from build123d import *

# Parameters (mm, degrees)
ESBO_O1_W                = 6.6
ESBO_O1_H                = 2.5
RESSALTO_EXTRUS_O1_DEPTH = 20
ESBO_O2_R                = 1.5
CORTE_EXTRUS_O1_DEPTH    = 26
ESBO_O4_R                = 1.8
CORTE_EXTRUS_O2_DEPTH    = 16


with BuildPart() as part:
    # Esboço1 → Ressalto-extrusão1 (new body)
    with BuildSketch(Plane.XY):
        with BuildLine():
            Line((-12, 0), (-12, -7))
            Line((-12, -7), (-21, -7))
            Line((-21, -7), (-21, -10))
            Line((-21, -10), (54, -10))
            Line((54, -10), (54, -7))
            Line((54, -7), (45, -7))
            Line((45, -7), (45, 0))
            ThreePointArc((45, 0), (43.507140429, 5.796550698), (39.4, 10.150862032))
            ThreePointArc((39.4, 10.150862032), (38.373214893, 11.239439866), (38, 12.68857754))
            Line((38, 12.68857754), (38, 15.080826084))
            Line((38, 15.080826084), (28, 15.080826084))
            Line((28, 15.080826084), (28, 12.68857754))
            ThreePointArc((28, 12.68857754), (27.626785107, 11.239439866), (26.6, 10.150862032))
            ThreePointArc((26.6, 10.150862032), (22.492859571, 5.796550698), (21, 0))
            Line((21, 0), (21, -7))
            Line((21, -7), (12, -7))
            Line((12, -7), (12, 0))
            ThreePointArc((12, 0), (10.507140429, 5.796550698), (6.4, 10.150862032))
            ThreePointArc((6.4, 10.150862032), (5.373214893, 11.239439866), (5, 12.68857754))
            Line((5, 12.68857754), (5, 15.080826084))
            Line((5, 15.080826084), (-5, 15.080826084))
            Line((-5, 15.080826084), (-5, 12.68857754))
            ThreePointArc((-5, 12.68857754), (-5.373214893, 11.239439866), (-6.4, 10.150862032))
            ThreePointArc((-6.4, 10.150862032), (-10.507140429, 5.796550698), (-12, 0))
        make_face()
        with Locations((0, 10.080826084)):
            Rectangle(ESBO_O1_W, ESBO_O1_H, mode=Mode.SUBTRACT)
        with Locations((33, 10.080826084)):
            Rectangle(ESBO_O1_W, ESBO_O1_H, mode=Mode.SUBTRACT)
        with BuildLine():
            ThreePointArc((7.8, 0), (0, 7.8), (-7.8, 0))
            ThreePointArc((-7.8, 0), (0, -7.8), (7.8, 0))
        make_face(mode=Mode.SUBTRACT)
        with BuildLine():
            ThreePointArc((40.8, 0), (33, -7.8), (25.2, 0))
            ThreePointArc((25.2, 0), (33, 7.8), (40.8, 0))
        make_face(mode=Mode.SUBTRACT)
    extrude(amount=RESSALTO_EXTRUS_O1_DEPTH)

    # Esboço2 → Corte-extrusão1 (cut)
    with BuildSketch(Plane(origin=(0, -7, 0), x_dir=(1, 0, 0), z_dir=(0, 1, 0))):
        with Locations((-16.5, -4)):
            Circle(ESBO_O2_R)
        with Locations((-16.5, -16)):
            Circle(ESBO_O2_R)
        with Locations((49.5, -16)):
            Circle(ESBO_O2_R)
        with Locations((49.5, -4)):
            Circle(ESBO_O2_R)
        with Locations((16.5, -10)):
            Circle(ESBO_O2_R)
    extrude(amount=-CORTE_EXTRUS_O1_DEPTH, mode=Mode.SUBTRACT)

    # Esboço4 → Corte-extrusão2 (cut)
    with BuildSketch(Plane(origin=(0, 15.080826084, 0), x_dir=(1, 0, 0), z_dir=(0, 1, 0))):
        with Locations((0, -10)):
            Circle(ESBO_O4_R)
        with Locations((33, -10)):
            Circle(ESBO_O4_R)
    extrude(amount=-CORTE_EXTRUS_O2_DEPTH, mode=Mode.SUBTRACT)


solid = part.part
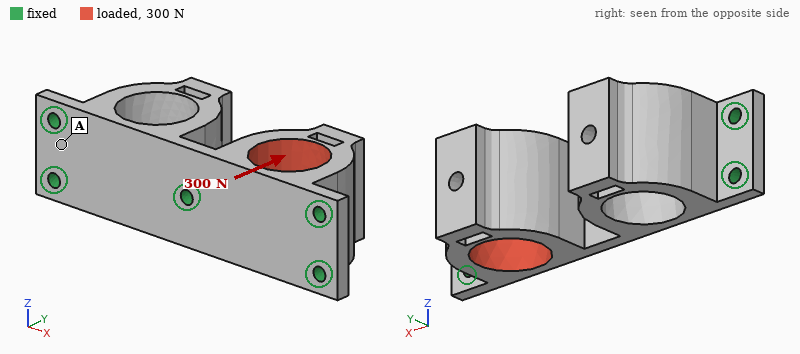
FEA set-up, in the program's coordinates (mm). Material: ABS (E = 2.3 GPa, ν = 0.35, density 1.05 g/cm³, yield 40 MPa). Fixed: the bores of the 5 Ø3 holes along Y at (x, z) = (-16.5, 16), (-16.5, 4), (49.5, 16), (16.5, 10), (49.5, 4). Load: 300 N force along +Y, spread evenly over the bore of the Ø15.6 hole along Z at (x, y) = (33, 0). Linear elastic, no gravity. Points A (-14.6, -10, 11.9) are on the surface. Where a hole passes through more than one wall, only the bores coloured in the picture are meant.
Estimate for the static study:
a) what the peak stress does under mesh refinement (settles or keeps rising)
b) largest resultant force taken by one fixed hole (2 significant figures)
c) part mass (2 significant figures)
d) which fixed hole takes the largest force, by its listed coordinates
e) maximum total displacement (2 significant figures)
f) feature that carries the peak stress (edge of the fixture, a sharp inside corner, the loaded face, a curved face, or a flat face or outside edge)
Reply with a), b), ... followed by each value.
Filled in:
a) keeps rising
b) 150 N
c) 14 g
d) (16.5, 10)
e) 0.11 mm
f) edge of the fixture
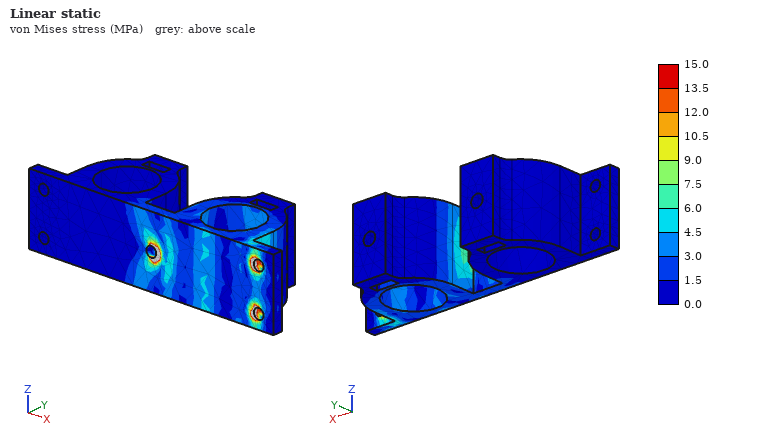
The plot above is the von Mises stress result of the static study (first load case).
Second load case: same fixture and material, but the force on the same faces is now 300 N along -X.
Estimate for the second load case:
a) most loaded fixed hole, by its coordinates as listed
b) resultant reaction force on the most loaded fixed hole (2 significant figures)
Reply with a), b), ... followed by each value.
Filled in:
a) (16.5, 10)
b) 150 N
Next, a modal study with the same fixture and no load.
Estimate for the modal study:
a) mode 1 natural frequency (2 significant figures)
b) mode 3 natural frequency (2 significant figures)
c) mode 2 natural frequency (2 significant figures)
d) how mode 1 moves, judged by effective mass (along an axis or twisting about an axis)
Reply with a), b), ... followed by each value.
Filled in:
a) 1800 Hz
b) 3200 Hz
c) 2000 Hz
d) along Z
